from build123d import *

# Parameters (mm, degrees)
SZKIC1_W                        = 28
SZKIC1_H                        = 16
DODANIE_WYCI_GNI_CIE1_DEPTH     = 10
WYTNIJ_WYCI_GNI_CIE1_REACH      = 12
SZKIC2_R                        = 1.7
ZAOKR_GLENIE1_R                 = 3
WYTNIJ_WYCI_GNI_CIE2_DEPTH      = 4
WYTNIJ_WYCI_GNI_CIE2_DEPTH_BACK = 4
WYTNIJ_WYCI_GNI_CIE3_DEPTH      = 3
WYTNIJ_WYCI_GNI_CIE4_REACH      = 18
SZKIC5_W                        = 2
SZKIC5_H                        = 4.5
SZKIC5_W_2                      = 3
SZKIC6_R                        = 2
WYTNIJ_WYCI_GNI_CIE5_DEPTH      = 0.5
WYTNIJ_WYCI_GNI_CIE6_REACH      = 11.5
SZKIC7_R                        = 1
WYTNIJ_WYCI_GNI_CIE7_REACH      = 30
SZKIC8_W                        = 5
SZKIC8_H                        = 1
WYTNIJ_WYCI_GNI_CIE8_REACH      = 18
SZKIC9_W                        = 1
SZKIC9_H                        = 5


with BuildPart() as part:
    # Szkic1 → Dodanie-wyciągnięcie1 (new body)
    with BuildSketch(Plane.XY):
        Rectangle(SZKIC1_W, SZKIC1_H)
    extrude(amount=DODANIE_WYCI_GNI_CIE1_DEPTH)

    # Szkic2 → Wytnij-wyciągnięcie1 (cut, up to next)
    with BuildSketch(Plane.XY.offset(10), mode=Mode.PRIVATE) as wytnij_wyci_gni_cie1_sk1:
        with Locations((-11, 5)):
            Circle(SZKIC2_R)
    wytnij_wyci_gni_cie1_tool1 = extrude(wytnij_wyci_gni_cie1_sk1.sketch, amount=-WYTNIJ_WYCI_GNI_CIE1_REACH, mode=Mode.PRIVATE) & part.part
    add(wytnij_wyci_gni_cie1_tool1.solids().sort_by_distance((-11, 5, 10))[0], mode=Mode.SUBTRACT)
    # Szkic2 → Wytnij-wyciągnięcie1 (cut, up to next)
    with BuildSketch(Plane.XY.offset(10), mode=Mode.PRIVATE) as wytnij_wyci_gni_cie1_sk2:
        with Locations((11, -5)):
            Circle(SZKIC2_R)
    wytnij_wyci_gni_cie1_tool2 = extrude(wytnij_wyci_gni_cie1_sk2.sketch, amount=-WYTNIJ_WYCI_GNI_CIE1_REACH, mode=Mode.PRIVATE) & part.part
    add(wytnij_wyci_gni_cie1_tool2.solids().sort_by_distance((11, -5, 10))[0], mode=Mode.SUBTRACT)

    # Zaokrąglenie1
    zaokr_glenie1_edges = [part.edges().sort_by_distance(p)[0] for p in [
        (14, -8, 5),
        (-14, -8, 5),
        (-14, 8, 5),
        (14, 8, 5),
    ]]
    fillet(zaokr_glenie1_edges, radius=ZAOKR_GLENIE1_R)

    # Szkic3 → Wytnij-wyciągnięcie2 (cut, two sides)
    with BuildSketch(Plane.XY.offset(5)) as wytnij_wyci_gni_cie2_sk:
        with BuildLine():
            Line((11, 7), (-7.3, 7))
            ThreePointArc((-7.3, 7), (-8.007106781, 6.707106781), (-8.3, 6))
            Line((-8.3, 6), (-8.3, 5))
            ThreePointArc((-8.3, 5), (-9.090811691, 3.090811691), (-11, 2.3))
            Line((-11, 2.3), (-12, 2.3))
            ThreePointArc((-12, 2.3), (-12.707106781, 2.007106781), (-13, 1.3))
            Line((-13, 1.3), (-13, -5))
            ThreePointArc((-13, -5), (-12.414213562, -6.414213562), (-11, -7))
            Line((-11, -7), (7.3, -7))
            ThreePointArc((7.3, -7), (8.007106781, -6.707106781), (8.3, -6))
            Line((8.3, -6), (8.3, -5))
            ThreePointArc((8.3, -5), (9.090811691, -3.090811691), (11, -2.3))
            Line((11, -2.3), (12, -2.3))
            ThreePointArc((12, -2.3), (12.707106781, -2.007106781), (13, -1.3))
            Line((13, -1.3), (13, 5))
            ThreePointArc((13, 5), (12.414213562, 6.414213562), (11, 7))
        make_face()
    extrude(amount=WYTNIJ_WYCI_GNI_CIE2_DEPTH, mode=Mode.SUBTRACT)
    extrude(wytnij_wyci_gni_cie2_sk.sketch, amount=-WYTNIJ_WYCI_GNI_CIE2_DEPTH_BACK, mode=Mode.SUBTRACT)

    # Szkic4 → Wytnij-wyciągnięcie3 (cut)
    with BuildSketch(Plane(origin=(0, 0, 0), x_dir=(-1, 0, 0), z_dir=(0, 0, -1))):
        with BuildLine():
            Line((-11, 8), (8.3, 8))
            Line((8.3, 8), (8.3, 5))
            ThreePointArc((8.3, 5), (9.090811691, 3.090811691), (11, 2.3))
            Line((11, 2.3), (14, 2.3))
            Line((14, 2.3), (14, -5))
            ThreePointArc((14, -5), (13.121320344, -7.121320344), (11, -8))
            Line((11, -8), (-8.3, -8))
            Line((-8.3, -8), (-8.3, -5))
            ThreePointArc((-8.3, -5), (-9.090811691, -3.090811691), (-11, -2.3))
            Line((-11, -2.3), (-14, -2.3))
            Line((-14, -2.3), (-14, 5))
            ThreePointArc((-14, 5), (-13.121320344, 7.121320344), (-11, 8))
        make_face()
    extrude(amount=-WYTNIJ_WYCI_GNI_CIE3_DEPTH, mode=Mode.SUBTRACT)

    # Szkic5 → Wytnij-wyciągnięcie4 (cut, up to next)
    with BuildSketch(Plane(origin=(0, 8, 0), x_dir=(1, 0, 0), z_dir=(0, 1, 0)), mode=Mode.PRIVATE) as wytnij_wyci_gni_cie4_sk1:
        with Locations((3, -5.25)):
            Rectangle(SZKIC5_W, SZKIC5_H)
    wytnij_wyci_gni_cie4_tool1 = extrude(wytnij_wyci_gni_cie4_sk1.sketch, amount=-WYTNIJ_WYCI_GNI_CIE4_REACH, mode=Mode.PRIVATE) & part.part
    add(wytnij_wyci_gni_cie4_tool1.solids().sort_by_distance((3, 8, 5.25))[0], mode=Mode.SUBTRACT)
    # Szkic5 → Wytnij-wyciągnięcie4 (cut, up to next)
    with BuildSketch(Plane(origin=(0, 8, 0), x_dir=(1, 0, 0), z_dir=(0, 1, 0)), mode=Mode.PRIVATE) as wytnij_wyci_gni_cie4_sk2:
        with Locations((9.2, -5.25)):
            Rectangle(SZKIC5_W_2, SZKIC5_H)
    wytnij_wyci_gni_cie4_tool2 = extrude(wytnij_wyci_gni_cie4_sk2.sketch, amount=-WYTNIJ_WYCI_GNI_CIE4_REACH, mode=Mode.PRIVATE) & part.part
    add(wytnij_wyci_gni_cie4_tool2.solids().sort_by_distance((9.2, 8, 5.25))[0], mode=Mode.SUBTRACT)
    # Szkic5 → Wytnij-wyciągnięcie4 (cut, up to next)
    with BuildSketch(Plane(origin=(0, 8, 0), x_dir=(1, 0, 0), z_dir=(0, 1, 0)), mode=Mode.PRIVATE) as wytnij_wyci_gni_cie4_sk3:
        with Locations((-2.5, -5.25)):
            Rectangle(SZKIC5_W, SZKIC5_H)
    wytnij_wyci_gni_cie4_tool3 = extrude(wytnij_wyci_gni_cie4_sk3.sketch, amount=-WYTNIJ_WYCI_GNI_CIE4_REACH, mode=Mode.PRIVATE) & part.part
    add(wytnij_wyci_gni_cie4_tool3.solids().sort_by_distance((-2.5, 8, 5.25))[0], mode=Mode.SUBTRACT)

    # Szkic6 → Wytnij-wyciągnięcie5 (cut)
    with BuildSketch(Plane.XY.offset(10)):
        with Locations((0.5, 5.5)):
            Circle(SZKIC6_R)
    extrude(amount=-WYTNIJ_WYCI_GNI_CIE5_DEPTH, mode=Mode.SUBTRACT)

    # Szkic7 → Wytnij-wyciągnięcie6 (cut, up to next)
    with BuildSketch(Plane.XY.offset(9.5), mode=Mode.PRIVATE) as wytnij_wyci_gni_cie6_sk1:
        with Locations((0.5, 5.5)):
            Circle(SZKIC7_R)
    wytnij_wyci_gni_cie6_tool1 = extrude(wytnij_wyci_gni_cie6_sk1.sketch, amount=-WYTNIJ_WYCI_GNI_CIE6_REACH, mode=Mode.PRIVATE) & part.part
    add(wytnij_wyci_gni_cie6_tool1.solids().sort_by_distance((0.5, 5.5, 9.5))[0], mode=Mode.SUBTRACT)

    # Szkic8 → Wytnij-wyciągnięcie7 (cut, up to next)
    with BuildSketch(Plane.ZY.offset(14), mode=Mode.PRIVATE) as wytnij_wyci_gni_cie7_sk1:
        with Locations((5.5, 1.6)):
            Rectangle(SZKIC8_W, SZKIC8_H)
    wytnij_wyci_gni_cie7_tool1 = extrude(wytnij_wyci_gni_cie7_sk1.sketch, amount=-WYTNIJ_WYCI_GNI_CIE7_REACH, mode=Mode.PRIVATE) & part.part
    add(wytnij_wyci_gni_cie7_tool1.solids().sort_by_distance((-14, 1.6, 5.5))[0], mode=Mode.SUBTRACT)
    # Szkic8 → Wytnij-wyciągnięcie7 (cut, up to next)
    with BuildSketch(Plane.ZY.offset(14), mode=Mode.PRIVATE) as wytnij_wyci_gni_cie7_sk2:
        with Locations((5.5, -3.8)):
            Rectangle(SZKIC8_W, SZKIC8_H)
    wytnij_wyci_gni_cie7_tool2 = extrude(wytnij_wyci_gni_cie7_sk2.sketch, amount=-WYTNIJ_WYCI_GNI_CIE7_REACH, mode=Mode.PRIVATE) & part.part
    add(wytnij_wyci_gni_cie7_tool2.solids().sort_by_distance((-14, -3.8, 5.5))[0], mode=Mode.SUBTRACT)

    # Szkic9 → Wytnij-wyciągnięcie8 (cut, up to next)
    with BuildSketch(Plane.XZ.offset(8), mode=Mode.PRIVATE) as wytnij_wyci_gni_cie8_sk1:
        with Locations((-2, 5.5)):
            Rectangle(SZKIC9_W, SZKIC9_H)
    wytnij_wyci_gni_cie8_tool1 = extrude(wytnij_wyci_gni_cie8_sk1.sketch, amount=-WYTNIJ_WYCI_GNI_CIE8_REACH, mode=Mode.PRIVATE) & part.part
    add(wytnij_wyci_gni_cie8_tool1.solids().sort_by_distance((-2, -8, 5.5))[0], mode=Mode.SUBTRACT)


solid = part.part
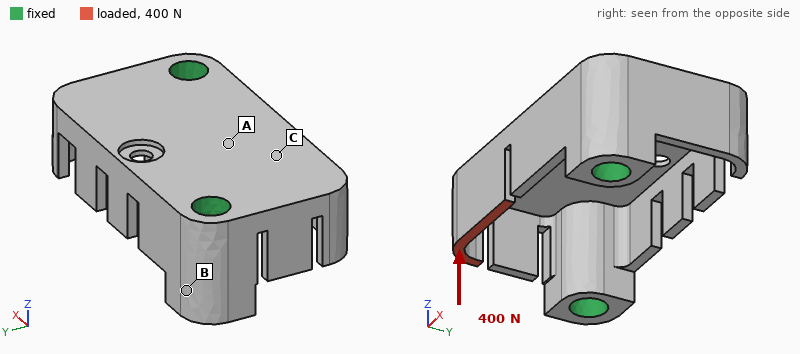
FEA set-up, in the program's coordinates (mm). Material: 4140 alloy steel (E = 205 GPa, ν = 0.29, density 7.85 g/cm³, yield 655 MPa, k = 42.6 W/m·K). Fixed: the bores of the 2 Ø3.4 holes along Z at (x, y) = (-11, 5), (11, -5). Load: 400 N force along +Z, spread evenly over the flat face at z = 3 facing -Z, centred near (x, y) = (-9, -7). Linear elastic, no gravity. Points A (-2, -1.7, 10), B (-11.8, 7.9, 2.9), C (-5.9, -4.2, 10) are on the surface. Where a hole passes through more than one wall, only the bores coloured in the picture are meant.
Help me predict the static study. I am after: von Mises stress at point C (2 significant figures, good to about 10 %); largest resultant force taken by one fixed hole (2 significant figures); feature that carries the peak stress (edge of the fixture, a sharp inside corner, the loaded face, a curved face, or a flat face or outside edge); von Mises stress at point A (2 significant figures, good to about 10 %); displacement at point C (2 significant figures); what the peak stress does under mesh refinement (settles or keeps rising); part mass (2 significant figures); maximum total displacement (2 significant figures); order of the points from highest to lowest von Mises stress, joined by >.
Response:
190 MPa
380 N
a sharp inside corner
100 MPa
0.032 mm
keeps rising
8.6 g
0.16 mm
C > A > B
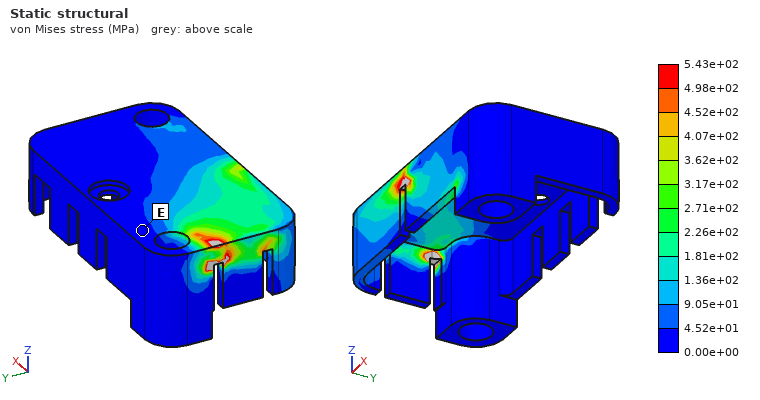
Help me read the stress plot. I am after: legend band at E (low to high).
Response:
0.00e+00 to 4.52e+01 MPa
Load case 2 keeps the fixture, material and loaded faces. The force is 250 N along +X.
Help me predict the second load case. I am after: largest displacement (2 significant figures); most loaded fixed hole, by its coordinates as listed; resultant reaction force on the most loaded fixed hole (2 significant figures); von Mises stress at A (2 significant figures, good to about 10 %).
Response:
100 µm
(11, -5)
240 N
48 MPa
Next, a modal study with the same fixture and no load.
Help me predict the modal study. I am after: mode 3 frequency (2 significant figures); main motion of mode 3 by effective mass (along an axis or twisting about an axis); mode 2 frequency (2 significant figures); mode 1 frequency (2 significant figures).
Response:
16 kHz
along Z
15 kHz
9100 Hz
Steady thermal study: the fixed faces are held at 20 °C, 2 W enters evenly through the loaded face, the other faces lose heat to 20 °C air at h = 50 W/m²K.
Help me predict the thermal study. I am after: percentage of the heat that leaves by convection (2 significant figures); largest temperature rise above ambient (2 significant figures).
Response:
29 %
41 K
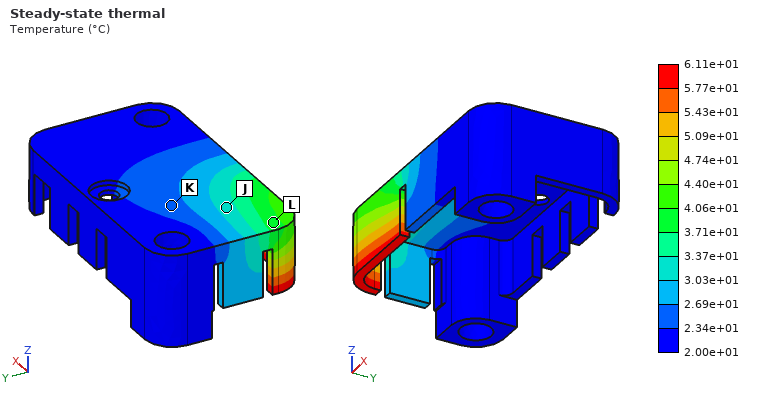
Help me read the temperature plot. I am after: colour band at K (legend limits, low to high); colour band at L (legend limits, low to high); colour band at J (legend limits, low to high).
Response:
2.34e+01 to 2.69e+01 °C
3.71e+01 to 4.06e+01 °C
3.03e+01 to 3.37e+01 °C
